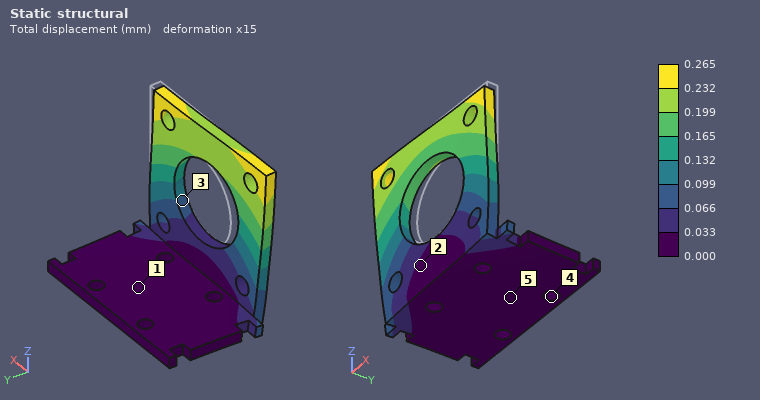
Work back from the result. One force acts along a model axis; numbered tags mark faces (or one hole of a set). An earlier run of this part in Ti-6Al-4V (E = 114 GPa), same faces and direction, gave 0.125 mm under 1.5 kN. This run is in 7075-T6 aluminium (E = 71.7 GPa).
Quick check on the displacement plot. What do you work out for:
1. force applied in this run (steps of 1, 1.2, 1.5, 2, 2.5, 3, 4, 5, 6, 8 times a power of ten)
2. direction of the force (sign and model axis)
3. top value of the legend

2 kN
-X
0.265 mm
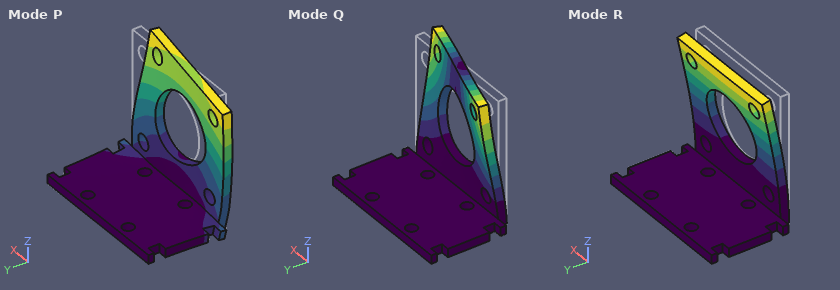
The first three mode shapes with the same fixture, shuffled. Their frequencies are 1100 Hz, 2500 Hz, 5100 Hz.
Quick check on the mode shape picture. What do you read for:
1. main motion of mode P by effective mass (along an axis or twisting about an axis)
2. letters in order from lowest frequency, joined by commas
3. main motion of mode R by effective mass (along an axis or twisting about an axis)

along X
R, Q, P
along Y
